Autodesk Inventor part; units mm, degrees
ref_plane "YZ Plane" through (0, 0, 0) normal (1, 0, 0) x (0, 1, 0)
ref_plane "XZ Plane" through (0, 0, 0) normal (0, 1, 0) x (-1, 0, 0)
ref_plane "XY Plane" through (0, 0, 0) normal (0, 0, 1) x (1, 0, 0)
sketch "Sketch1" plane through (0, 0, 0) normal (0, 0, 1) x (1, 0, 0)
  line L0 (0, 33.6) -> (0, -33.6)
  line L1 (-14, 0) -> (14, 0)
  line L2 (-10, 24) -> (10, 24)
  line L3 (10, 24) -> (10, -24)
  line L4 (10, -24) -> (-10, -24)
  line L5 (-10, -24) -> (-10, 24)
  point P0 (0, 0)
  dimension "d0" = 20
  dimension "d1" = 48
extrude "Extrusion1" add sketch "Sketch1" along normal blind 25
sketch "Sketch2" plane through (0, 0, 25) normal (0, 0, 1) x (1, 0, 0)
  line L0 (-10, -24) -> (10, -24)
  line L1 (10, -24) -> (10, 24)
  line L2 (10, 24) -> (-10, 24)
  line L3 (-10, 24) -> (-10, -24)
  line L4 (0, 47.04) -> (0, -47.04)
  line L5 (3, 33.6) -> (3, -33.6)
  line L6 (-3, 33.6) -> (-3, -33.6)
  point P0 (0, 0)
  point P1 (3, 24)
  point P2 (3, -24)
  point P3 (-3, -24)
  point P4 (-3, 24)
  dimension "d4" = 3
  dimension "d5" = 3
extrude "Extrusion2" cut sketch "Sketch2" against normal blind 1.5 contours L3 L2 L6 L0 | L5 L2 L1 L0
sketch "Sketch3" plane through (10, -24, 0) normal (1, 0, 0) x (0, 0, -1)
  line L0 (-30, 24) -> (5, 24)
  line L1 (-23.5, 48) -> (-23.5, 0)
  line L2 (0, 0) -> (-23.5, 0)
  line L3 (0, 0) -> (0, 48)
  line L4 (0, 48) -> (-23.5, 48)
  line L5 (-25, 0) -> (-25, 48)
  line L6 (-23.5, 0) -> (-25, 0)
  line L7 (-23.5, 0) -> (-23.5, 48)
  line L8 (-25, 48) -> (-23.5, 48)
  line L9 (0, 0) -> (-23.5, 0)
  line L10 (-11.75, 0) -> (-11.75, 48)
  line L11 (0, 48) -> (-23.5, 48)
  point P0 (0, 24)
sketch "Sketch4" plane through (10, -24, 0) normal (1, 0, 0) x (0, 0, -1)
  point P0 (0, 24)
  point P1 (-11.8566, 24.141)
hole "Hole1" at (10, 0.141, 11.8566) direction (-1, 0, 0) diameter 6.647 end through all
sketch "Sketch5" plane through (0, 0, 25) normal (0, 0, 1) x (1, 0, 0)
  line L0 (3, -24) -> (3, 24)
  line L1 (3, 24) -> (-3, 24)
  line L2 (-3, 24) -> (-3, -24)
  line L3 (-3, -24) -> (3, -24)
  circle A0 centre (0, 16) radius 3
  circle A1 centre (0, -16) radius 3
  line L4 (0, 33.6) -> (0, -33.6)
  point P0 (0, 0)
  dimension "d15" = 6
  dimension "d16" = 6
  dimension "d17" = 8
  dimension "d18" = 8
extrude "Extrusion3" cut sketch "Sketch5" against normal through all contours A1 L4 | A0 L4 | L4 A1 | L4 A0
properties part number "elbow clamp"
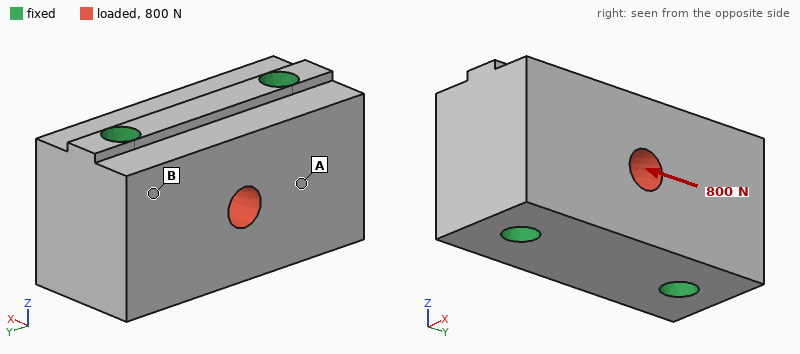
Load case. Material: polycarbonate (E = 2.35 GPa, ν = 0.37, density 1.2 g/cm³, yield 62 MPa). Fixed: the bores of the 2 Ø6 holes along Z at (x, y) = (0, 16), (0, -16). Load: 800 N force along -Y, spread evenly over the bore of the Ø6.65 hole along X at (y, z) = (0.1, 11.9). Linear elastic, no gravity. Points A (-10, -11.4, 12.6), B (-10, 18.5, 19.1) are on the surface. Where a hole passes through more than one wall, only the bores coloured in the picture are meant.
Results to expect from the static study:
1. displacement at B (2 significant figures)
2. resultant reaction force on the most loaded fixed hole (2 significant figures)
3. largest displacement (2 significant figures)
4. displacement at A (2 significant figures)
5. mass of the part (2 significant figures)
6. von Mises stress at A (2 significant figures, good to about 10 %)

2.5 µm
400 N
9.2 µm
4.3 µm
25 g
0.82 MPa
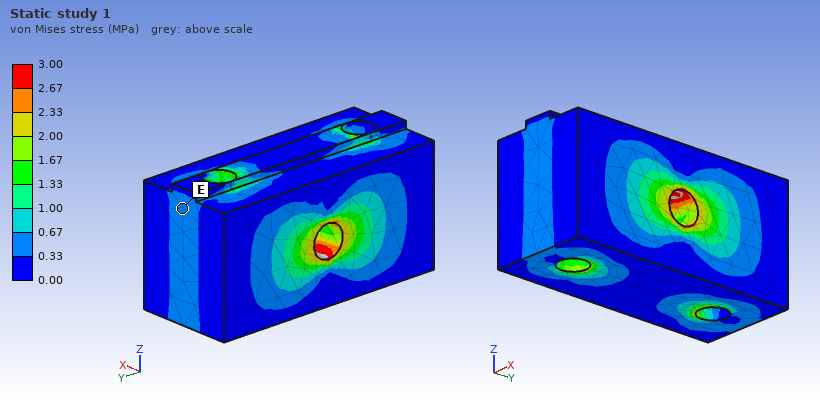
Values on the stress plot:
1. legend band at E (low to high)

0.33 to 0.67 MPa
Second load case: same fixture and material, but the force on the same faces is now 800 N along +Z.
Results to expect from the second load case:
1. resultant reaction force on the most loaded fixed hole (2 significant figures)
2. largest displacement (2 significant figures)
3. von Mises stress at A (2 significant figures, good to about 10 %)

400 N
20 µm
1.2 MPa
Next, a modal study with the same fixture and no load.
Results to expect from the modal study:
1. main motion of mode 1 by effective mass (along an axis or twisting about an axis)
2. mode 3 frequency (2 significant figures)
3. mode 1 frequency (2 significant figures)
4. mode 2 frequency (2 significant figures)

along X
13 kHz
11 kHz
12 kHz
